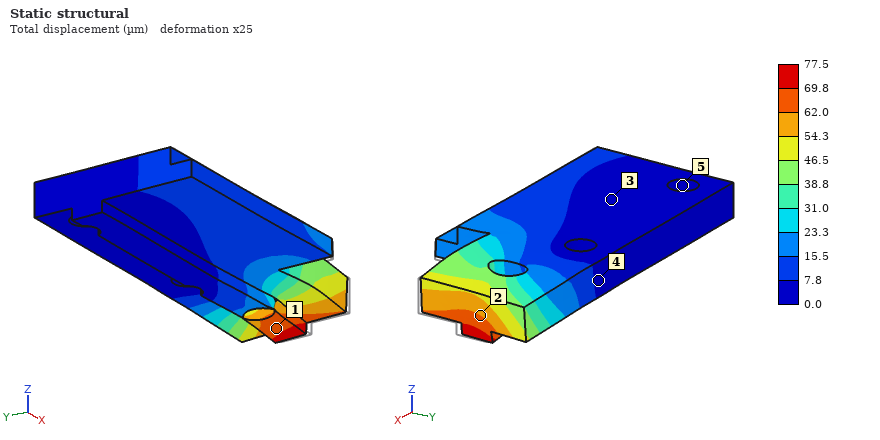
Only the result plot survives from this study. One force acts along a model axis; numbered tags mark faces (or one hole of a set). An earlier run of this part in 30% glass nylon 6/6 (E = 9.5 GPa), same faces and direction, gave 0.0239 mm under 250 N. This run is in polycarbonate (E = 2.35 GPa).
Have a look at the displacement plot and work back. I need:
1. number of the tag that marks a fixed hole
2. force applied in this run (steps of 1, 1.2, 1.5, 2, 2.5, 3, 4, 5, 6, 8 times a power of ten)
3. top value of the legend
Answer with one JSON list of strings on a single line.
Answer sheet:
["5", "200 N", "77.5 µm"]
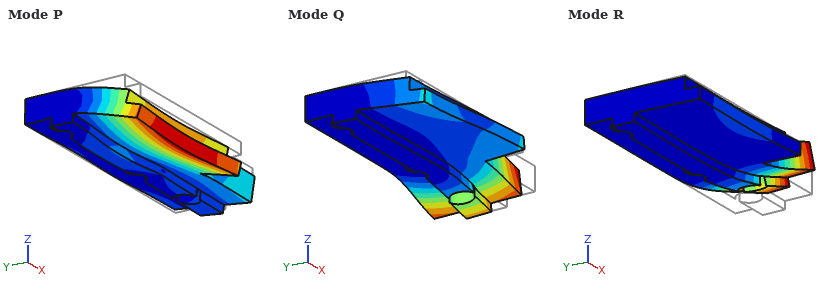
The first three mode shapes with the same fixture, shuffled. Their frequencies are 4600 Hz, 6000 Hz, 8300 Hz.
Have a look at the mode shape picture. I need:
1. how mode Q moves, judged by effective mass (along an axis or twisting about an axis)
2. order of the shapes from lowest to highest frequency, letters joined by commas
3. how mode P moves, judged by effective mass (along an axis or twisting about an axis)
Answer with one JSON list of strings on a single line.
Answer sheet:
["along Y", "R, P, Q", "along Z"]
